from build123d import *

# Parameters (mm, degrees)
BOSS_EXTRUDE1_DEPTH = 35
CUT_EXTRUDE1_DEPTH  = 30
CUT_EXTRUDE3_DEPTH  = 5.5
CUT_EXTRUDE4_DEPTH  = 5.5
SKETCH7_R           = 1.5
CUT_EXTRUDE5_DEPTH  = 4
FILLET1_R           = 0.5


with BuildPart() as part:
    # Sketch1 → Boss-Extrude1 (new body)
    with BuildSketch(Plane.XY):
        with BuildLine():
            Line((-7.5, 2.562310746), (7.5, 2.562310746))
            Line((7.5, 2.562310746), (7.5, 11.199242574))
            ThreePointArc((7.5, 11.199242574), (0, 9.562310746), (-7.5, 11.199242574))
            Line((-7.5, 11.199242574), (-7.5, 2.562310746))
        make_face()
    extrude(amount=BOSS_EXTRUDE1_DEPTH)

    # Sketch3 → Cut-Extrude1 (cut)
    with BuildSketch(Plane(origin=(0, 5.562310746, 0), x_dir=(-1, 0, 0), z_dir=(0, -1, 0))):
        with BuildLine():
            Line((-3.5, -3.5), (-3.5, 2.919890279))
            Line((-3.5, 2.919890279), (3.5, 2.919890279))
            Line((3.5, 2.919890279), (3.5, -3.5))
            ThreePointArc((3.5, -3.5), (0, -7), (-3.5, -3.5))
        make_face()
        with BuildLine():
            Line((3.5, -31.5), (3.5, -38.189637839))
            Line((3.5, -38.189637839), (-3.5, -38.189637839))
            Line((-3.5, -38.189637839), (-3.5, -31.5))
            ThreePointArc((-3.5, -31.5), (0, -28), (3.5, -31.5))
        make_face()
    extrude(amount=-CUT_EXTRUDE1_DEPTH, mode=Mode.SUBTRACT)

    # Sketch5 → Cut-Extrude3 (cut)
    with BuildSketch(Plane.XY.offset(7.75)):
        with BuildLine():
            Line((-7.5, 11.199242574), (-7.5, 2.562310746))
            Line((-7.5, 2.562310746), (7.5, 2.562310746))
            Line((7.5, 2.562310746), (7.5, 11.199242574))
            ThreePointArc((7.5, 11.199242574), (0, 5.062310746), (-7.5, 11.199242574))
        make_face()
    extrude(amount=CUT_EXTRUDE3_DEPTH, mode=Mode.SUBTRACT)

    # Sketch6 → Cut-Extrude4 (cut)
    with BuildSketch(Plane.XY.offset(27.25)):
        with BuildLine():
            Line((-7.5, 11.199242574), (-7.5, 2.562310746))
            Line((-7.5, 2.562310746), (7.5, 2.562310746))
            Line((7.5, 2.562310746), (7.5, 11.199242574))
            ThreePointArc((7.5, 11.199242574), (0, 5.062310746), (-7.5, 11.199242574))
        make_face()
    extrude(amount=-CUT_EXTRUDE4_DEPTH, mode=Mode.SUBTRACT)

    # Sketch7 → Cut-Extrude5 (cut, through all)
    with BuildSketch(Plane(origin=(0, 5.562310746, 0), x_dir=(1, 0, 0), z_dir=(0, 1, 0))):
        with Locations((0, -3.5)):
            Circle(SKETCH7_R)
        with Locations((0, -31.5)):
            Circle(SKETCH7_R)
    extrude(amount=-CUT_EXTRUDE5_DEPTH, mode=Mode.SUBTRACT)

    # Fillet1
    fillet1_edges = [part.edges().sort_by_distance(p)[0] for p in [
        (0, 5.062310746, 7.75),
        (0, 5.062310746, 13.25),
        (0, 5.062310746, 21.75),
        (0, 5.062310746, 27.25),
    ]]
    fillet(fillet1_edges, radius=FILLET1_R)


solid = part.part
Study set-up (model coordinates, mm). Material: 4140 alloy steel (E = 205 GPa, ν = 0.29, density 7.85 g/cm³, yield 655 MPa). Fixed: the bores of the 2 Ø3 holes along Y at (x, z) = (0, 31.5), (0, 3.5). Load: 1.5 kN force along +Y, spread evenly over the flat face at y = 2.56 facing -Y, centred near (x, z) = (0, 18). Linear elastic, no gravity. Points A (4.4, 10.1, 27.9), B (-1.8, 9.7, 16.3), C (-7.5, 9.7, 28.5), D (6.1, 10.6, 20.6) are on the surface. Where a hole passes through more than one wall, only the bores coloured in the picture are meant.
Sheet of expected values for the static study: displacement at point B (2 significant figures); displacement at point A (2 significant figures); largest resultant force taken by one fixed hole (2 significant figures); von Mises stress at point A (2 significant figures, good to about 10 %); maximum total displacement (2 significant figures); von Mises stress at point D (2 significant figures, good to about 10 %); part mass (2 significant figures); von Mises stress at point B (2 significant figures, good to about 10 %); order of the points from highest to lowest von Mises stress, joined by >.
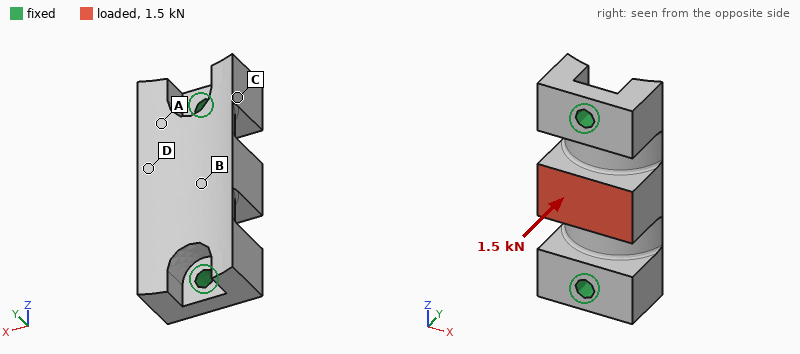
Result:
7.3 µm
3.0 µm
1.1 kN
21 MPa
8.2 µm
75 MPa
23 g
61 MPa
D > B > A > C
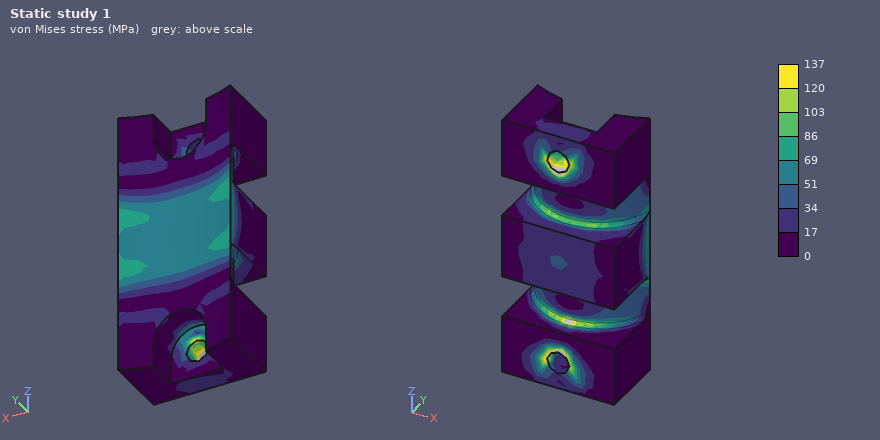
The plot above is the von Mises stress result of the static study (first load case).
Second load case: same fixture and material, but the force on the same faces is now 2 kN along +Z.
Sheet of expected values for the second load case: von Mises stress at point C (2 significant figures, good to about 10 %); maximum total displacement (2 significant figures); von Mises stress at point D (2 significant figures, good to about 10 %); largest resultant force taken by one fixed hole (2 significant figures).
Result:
20 MPa
11 µm
49 MPa
1.0 kN
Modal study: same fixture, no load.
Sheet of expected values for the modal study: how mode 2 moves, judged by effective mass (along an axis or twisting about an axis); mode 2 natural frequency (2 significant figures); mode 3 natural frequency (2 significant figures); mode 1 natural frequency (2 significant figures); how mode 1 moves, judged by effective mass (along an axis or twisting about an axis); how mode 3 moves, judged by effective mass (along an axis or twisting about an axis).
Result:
along Y
22 kHz
25 kHz
15 kHz
along X
along X
